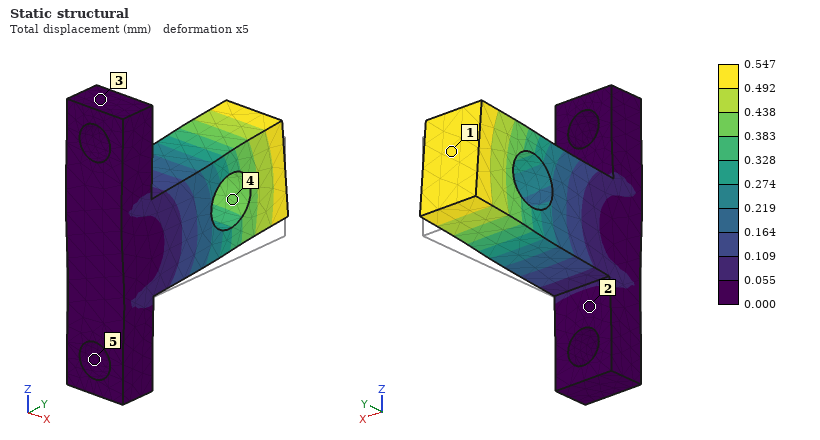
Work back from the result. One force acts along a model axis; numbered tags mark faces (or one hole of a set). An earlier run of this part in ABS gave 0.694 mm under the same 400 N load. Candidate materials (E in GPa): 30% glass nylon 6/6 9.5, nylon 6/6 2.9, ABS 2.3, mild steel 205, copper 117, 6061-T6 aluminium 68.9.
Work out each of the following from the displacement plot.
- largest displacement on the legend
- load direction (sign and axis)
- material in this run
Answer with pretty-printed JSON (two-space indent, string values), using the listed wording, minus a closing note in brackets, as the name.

{
  "largest displacement on the legend": "0.547 mm",
  "load direction": "+Z",
  "material in this run": "nylon 6/6"
}
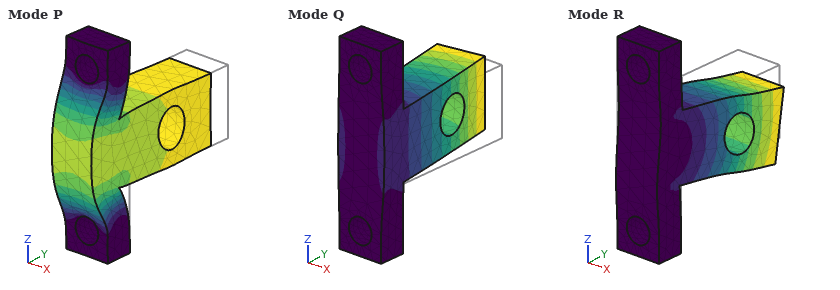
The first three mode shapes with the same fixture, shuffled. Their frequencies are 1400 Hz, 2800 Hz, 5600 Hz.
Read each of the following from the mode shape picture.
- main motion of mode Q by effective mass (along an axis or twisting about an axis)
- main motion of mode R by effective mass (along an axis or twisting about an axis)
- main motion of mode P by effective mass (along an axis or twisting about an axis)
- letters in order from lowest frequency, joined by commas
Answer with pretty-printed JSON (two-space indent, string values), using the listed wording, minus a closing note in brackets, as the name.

{
  "main motion of mode Q by effective mass": "along X",
  "main motion of mode R by effective mass": "along Z",
  "main motion of mode P by effective mass": "along Y",
  "letters in order from lowest frequency, joined by commas": "Q, R, P"
}
